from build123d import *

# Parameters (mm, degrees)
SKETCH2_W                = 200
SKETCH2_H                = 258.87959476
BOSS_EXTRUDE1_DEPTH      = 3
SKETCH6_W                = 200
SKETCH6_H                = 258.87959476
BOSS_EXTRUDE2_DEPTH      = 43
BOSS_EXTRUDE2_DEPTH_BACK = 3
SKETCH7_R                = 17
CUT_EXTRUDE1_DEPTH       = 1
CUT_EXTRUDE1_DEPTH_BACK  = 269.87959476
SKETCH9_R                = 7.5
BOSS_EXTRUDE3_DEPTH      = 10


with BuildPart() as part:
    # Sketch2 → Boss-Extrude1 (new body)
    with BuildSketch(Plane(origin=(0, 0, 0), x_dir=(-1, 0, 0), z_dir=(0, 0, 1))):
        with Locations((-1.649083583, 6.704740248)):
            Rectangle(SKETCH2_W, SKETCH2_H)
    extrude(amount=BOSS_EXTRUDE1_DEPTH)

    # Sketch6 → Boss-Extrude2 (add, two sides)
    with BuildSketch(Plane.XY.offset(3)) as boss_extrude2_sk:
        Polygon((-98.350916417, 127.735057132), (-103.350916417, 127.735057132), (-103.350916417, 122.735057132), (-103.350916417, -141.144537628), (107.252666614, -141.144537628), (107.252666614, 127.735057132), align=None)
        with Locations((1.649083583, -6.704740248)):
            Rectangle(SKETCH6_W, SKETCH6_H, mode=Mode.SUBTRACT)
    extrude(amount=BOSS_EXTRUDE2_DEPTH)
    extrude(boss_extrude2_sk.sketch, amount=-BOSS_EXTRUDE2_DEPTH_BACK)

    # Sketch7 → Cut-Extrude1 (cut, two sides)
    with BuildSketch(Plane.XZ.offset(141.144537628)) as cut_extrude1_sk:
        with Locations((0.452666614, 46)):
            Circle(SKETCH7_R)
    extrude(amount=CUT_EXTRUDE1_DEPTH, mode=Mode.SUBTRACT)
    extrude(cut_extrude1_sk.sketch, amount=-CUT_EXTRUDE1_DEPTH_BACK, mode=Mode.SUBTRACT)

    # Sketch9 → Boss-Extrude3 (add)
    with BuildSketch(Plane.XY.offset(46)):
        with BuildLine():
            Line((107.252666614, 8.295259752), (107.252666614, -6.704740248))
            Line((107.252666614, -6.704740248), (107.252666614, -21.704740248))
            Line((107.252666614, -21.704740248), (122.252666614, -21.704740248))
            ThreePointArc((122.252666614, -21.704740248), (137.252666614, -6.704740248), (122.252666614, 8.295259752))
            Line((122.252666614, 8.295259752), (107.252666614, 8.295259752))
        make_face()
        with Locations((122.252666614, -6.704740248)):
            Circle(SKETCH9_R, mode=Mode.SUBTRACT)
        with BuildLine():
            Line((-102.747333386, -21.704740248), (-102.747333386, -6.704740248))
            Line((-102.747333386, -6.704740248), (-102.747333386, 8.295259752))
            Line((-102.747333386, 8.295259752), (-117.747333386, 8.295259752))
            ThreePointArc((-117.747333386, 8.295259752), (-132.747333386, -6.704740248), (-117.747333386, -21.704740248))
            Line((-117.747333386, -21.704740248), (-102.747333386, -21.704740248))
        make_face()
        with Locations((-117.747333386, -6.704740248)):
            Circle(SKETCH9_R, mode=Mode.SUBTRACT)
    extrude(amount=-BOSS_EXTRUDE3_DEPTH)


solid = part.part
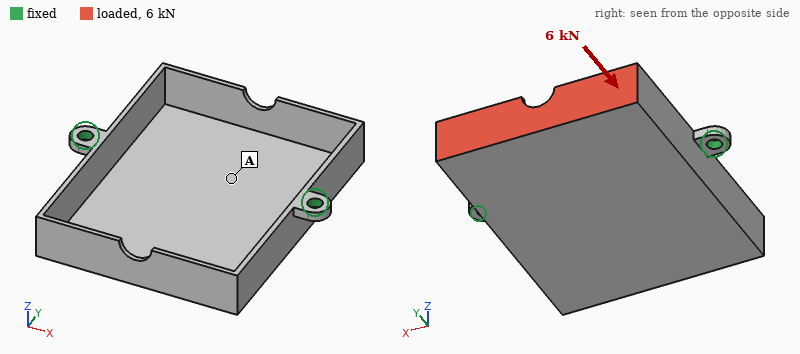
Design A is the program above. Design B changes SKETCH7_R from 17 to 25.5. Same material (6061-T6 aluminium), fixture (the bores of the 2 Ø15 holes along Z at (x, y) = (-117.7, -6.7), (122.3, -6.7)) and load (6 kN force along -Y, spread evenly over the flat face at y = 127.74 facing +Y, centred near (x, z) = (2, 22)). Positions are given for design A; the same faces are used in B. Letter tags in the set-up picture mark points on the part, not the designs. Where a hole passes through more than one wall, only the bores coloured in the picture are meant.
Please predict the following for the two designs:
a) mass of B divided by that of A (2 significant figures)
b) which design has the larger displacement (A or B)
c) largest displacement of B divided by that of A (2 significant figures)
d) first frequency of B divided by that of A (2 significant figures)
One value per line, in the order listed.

0.99
A
0.87
1.0
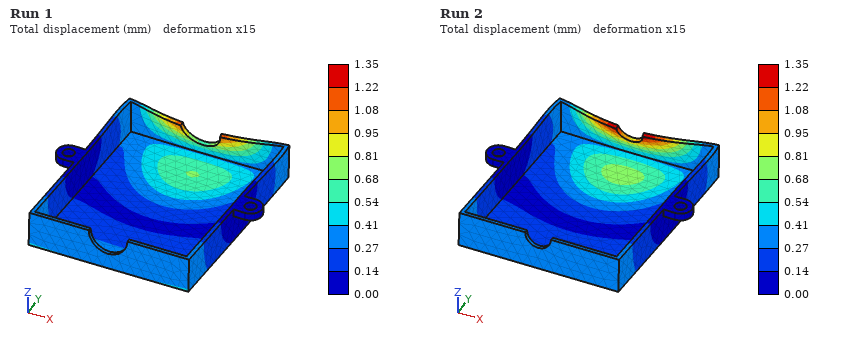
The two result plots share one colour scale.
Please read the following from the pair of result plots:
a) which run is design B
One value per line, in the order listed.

Run 1
